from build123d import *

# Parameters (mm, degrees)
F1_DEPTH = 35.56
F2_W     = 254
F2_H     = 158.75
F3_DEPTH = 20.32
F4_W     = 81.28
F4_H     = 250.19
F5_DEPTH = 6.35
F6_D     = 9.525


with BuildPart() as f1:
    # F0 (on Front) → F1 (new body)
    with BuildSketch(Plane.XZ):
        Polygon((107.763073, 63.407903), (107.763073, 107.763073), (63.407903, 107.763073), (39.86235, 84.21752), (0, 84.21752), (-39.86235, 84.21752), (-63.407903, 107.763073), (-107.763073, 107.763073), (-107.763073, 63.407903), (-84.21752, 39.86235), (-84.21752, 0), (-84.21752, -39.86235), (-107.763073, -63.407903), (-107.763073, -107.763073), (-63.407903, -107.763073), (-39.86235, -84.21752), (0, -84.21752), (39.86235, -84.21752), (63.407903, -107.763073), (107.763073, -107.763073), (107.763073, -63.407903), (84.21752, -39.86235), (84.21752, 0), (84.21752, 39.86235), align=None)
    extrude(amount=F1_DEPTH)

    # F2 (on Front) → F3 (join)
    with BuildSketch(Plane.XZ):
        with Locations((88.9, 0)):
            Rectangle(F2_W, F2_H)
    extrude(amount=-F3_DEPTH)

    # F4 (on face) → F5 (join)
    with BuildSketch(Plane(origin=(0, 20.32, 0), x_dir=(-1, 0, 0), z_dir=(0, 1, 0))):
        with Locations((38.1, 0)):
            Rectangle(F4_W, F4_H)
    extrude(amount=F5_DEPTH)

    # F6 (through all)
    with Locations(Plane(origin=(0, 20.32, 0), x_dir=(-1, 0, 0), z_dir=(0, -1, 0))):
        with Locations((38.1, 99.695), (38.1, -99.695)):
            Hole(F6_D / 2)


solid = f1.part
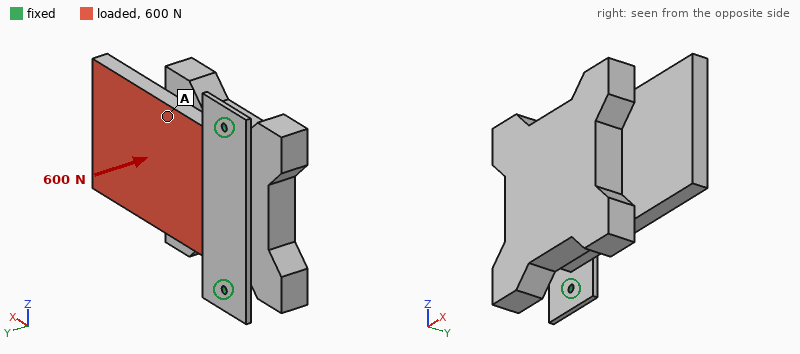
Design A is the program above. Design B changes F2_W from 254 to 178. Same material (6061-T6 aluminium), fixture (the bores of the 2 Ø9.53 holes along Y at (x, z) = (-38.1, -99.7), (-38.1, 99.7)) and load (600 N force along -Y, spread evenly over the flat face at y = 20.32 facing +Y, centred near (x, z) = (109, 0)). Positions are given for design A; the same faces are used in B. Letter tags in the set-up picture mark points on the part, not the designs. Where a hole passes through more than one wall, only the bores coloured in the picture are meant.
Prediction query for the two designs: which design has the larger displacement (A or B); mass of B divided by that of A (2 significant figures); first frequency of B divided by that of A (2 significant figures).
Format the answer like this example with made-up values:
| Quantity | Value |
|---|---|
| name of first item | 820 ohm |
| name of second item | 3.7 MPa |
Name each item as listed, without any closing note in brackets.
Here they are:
| Quantity | Value |
|---|---|
| which design has the larger displacement | B |
| mass of B divided by that of A | 0.89 |
| first frequency of B divided by that of A | 0.69 |
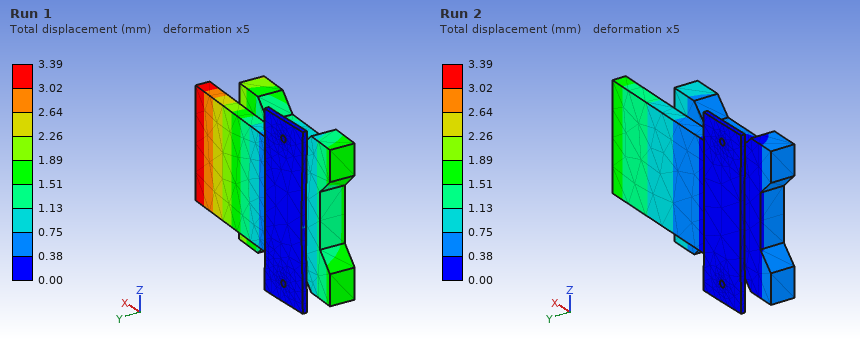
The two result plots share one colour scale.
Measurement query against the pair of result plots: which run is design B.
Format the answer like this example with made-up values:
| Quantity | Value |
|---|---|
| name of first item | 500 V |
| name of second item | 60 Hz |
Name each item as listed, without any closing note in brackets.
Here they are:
| Quantity | Value |
|---|---|
| which run is design B | Run 1 |
